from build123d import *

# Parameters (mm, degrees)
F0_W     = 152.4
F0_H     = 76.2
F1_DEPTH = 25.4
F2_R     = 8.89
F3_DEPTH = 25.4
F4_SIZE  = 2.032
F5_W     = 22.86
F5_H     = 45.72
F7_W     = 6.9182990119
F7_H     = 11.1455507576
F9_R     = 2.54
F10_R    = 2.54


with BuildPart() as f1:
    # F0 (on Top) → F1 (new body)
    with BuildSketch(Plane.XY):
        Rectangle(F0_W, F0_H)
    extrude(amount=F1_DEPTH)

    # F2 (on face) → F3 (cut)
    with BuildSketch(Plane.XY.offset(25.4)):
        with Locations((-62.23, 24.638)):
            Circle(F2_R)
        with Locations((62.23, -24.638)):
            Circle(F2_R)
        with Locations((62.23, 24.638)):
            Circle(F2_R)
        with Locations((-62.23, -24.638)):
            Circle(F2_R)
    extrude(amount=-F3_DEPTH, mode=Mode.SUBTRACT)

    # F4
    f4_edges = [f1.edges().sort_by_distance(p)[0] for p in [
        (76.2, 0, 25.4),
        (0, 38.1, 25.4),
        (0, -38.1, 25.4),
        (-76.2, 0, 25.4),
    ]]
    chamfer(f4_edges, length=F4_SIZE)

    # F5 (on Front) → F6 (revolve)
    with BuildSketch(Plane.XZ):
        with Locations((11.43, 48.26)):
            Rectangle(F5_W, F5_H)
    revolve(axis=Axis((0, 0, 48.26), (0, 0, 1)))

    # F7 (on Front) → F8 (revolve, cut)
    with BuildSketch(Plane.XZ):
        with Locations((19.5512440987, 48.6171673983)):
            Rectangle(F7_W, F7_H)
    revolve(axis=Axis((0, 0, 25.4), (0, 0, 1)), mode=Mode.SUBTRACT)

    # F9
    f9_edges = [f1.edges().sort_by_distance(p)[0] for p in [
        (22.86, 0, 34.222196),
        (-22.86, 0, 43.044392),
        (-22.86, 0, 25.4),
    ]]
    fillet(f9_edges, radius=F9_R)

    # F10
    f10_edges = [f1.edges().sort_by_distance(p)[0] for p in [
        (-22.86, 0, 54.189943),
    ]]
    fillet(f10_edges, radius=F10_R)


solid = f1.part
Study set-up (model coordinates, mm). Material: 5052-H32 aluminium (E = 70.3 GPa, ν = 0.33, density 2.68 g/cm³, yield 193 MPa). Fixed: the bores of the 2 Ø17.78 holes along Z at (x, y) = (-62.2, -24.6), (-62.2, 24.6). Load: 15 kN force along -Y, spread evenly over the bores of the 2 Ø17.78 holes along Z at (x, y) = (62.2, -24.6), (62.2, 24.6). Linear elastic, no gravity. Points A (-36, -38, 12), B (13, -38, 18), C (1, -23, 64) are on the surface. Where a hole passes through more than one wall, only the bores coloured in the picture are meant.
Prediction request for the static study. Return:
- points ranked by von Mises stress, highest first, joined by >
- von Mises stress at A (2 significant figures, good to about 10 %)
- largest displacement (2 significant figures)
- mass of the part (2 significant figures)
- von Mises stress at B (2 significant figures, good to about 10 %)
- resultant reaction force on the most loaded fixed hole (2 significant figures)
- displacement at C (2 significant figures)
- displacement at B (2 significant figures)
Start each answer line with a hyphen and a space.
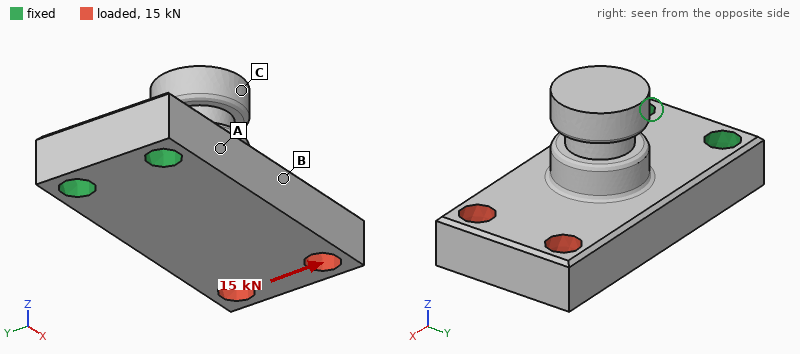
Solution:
- A > B > C
- 56 MPa
- 0.21 mm
- 900 g
- 30 MPa
- 33 kN
- 0.057 mm
- 0.094 mm
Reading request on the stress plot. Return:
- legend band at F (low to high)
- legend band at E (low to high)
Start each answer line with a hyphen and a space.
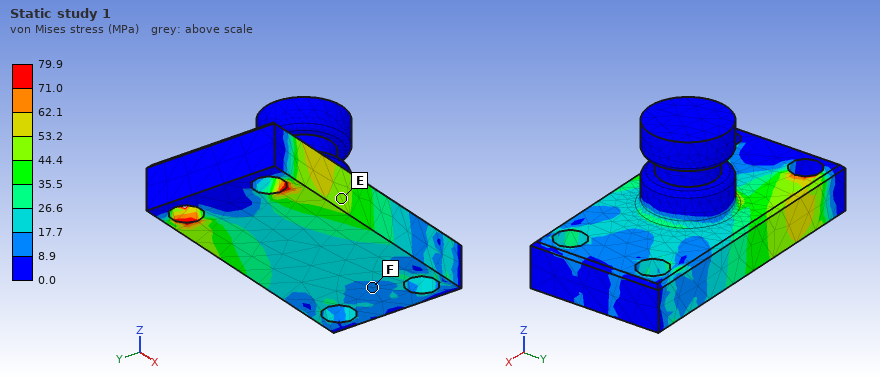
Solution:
- 8.9 to 17.7 MPa
- 44.4 to 53.2 MPa
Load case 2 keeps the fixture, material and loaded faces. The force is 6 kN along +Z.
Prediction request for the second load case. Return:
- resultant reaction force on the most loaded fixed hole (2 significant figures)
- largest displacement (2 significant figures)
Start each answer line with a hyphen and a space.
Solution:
- 3.0 kN
- 0.52 mm
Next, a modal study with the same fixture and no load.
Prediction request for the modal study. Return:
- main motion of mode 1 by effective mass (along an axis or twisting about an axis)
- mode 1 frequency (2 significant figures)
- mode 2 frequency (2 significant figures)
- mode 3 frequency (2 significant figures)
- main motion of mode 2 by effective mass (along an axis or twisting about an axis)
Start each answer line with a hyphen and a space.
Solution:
- along Z
- 1200 Hz
- 2900 Hz
- 3400 Hz
- along Y
